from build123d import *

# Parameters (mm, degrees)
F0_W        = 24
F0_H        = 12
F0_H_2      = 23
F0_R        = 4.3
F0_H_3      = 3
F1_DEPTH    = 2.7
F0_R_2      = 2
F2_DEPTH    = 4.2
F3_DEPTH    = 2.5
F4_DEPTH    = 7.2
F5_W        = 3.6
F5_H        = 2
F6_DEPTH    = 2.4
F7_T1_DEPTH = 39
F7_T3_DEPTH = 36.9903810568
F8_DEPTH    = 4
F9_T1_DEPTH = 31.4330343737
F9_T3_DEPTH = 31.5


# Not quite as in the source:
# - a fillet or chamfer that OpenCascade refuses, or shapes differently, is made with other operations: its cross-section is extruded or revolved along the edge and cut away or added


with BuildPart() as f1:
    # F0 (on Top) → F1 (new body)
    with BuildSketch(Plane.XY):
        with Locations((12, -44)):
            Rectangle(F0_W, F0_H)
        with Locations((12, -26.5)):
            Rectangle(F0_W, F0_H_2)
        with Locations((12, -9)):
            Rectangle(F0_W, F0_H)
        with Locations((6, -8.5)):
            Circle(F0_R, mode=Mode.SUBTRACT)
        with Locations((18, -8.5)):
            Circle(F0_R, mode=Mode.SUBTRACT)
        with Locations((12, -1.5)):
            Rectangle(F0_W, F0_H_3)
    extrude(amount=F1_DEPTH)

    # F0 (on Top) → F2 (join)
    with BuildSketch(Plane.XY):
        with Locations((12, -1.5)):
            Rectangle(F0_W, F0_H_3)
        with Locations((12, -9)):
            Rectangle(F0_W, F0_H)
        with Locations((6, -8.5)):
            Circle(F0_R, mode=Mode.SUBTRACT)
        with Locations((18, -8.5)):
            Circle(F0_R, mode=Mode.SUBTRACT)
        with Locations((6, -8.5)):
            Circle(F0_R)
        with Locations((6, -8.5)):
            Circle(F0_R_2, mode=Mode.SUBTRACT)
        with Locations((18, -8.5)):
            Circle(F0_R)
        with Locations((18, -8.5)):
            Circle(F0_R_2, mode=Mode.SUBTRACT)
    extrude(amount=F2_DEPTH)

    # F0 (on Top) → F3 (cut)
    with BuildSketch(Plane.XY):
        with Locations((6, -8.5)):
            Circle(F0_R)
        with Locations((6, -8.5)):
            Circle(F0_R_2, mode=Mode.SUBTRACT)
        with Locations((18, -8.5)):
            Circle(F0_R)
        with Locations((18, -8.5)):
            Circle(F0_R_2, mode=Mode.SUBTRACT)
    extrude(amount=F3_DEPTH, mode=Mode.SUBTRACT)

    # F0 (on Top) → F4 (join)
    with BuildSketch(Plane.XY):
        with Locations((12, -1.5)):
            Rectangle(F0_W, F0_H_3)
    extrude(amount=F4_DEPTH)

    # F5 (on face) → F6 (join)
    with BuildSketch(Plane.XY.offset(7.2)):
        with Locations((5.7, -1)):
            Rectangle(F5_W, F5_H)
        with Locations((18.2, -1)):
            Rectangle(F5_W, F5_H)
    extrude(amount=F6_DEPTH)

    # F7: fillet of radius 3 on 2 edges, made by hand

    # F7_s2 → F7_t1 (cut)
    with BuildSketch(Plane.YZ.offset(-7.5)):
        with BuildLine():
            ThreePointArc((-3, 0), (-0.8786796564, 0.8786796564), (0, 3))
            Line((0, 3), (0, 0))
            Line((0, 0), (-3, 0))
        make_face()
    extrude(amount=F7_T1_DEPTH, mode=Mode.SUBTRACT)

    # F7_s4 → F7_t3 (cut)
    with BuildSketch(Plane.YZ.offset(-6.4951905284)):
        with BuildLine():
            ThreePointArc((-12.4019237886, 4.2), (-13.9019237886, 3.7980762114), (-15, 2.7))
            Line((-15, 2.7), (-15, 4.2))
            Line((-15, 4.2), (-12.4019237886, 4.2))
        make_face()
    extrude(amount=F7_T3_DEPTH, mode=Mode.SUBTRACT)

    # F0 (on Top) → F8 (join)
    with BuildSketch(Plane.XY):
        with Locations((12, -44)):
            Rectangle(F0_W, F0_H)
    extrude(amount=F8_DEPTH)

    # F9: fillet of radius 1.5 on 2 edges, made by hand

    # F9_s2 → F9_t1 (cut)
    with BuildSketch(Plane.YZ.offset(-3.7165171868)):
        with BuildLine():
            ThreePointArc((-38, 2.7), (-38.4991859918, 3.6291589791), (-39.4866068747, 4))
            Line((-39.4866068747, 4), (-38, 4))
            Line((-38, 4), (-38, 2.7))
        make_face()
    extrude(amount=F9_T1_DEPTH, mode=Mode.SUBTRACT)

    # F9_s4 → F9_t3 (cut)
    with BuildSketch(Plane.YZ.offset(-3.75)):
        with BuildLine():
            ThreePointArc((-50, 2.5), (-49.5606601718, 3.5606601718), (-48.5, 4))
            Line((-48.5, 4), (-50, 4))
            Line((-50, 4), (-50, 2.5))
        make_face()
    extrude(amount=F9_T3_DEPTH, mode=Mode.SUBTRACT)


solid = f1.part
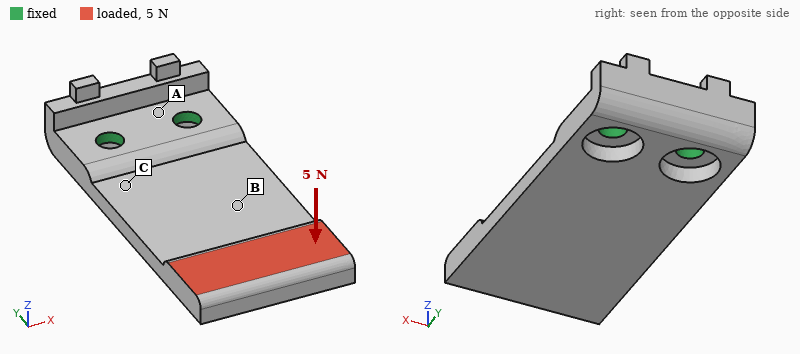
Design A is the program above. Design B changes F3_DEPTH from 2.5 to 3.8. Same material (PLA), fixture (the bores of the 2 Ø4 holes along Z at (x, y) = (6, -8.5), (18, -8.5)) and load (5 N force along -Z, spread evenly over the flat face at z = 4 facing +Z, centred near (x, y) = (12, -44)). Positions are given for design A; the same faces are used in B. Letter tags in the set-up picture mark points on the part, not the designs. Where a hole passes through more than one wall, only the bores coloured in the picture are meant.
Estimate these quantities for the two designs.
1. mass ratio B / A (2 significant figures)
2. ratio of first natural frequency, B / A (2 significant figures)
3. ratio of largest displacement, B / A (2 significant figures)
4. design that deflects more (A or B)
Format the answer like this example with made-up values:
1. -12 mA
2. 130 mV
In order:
1. 0.97
2. 0.49
3. 3.6
4. B
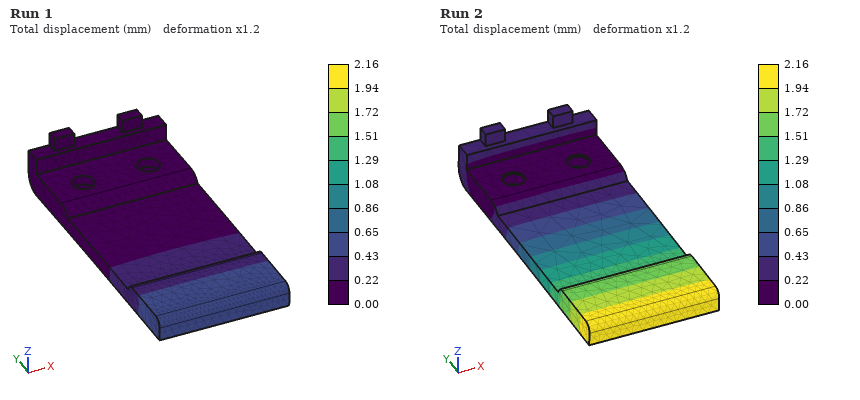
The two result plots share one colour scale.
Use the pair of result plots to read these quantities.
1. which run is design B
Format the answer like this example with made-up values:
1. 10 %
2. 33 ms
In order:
1. Run 2
